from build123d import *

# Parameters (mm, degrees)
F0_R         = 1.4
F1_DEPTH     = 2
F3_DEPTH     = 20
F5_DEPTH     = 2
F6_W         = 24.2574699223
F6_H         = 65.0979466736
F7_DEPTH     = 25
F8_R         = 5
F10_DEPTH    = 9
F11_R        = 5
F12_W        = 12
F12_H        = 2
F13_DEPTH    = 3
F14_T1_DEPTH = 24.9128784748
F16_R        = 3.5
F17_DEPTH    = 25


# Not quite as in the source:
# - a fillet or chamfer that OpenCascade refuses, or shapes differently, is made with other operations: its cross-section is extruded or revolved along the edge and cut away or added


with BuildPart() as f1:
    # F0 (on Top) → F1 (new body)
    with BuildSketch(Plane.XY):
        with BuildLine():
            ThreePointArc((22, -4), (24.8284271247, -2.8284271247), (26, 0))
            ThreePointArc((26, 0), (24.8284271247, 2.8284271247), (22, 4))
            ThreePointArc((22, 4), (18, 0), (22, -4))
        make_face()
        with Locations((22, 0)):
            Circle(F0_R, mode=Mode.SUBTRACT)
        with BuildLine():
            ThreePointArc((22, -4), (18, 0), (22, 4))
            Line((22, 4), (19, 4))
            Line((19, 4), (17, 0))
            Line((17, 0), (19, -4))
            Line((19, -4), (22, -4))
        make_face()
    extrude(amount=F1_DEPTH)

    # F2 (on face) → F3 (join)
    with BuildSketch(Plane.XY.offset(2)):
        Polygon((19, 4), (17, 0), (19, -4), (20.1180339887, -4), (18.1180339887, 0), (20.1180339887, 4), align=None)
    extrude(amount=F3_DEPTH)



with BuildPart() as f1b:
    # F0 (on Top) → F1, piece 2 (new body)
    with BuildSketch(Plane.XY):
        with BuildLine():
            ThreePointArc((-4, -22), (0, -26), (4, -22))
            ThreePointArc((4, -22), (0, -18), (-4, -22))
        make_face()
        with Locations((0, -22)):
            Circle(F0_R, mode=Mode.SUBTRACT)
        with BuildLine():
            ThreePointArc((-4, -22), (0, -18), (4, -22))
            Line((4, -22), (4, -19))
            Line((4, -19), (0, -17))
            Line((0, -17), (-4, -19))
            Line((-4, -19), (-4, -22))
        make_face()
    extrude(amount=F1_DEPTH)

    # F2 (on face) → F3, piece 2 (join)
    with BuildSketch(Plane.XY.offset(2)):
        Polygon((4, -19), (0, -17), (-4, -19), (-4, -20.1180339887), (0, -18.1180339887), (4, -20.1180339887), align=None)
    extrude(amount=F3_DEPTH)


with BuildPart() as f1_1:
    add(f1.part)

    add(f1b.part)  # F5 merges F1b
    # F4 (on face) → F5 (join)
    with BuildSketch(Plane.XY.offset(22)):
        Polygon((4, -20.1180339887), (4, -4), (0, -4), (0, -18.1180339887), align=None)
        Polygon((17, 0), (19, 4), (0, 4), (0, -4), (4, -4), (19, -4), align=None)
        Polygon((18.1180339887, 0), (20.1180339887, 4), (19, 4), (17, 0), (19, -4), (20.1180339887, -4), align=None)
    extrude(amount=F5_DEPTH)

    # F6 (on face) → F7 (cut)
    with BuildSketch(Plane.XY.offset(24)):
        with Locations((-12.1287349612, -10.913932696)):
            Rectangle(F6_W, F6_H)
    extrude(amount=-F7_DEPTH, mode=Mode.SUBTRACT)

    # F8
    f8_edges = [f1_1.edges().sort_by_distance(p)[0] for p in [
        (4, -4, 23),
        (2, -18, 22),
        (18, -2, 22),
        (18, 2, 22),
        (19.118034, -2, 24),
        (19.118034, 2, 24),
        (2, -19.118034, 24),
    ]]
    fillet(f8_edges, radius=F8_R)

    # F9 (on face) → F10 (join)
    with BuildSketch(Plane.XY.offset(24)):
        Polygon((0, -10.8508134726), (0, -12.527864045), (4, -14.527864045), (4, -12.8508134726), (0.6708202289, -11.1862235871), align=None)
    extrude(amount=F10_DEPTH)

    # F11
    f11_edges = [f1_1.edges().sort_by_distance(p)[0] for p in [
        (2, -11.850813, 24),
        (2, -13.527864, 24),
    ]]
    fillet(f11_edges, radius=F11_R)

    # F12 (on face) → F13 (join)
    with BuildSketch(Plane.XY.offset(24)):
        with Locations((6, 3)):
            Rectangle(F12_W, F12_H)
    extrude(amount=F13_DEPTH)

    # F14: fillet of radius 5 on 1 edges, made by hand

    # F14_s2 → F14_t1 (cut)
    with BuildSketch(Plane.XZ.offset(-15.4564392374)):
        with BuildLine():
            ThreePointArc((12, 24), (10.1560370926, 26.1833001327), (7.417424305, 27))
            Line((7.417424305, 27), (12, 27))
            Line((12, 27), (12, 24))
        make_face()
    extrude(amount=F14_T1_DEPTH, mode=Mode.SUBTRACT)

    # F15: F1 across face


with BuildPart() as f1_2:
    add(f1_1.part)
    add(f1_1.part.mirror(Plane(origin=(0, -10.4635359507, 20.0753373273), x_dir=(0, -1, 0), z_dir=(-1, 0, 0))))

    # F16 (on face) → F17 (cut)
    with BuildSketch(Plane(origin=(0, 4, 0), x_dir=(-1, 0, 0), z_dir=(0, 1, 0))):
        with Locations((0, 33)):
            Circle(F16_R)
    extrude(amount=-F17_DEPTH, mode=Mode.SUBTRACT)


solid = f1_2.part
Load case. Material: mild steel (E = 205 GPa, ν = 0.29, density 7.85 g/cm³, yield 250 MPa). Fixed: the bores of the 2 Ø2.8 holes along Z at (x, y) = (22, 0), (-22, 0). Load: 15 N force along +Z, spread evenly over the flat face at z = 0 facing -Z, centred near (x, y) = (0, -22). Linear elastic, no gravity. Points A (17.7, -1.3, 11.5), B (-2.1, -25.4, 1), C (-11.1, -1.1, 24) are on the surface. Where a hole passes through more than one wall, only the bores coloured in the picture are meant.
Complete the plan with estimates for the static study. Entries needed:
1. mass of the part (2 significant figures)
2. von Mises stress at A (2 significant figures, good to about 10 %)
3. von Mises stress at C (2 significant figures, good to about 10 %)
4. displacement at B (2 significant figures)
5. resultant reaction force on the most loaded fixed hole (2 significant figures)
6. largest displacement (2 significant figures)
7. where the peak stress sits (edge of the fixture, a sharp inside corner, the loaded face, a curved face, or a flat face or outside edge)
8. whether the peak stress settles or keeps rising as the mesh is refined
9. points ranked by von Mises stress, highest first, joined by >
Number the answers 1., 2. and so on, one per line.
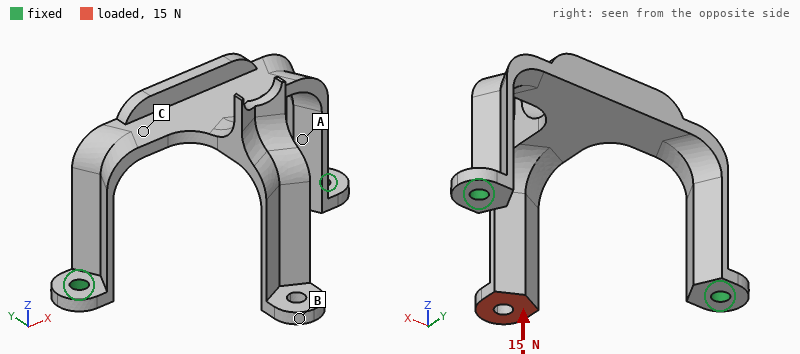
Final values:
1. 16 g
2. 11 MPa
3. 28 MPa
4. 0.11 mm
5. 8.2 N
6. 0.12 mm
7. edge of the fixture
8. keeps rising
9. C > A > B
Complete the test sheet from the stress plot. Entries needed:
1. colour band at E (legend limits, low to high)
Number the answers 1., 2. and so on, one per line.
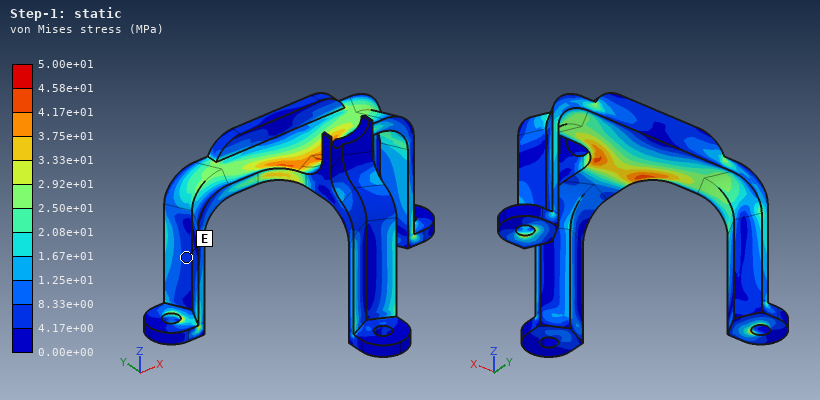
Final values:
1. 4.17e+00 to 8.33e+00 MPa
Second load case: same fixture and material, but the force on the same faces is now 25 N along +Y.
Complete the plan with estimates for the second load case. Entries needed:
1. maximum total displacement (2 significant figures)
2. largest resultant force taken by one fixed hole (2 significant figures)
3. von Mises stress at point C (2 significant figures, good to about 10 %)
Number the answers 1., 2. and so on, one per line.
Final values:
1. 0.30 mm
2. 13 N
3. 44 MPa
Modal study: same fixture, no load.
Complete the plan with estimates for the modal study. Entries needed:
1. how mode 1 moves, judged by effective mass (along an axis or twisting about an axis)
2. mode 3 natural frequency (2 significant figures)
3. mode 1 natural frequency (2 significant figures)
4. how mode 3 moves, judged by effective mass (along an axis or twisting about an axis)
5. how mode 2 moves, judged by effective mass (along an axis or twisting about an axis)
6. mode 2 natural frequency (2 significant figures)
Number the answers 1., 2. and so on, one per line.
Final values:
1. along Z
2. 2100 Hz
3. 1100 Hz
4. along Y
5. along X
6. 1400 Hz
